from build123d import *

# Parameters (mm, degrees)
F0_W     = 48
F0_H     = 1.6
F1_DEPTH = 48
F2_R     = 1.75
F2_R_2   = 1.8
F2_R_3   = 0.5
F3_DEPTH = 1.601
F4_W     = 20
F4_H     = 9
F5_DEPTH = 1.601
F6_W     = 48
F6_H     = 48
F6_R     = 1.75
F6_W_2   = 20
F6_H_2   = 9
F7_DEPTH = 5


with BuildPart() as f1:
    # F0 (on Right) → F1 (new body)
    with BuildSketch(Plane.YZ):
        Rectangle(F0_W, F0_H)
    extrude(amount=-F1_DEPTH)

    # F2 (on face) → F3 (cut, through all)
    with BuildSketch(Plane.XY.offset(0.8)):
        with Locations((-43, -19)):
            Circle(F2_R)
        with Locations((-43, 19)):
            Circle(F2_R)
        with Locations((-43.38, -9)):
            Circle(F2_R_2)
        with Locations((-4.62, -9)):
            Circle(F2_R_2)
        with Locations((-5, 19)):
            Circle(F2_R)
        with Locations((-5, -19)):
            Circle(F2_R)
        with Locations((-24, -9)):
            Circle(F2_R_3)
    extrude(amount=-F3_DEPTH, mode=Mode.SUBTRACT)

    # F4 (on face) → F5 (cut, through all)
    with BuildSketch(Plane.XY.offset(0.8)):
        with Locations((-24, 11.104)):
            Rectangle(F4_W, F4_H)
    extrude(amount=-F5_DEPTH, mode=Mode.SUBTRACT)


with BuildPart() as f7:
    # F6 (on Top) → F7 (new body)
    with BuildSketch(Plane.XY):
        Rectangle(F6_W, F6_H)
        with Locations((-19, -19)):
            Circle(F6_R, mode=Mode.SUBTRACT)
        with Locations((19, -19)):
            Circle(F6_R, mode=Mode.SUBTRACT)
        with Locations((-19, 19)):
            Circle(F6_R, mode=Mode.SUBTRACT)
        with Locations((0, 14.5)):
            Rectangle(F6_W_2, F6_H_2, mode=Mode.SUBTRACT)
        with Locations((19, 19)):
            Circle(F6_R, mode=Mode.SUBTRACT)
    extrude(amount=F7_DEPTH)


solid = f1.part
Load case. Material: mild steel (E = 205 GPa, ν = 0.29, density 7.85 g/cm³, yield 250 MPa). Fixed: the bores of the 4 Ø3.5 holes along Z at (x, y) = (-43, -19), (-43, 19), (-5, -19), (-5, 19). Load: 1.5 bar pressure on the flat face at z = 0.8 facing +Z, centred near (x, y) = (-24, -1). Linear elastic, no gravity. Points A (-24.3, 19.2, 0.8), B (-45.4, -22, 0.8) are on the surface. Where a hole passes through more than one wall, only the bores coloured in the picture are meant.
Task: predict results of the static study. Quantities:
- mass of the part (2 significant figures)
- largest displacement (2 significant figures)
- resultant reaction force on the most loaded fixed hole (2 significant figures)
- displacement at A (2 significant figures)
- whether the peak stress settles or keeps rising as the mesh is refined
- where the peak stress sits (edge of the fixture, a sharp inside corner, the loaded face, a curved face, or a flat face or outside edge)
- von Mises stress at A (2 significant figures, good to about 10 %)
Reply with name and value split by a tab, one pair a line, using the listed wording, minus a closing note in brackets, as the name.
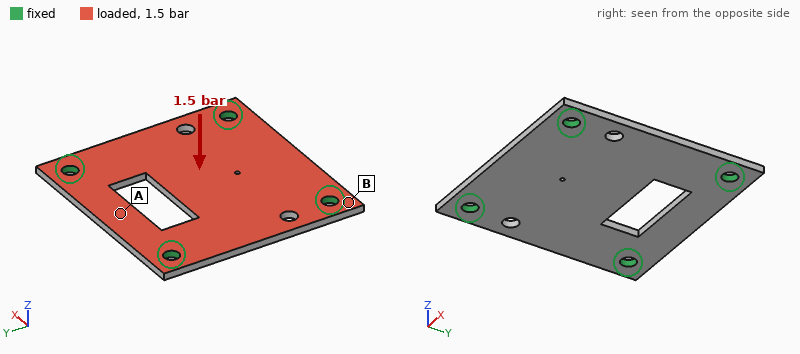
mass of the part	26 g
largest displacement	28 µm
resultant reaction force on the most loaded fixed hole	81 N
displacement at A	10 µm
whether the peak stress settles or keeps rising as the mesh is refined	keeps rising
where the peak stress sits	edge of the fixture
von Mises stress at A	19 MPa
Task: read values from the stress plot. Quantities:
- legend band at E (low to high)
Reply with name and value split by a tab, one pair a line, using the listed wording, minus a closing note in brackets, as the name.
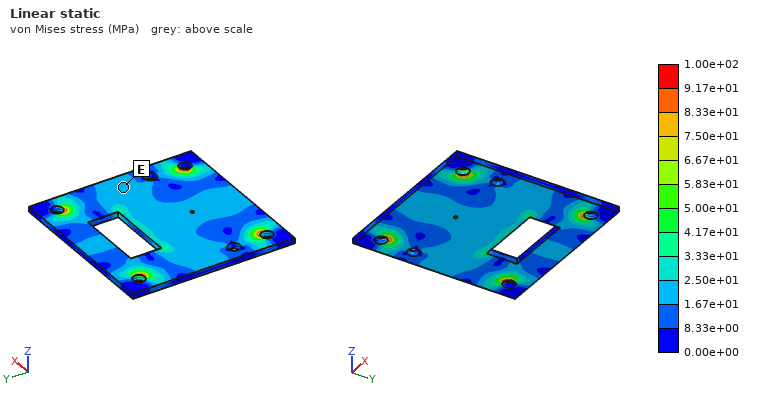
legend band at E	1.67e+01 to 2.50e+01 MPa
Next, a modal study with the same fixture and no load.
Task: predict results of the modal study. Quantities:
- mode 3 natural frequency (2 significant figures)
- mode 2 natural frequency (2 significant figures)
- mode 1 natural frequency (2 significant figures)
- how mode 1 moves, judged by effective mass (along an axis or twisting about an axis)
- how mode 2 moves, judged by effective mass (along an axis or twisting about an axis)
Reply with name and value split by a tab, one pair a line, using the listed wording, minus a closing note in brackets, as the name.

mode 3 natural frequency	7100 Hz
mode 2 natural frequency	6800 Hz
mode 1 natural frequency	4200 Hz
how mode 1 moves, judged by effective mass	along Z
how mode 2 moves, judged by effective mass	twisting about Y
